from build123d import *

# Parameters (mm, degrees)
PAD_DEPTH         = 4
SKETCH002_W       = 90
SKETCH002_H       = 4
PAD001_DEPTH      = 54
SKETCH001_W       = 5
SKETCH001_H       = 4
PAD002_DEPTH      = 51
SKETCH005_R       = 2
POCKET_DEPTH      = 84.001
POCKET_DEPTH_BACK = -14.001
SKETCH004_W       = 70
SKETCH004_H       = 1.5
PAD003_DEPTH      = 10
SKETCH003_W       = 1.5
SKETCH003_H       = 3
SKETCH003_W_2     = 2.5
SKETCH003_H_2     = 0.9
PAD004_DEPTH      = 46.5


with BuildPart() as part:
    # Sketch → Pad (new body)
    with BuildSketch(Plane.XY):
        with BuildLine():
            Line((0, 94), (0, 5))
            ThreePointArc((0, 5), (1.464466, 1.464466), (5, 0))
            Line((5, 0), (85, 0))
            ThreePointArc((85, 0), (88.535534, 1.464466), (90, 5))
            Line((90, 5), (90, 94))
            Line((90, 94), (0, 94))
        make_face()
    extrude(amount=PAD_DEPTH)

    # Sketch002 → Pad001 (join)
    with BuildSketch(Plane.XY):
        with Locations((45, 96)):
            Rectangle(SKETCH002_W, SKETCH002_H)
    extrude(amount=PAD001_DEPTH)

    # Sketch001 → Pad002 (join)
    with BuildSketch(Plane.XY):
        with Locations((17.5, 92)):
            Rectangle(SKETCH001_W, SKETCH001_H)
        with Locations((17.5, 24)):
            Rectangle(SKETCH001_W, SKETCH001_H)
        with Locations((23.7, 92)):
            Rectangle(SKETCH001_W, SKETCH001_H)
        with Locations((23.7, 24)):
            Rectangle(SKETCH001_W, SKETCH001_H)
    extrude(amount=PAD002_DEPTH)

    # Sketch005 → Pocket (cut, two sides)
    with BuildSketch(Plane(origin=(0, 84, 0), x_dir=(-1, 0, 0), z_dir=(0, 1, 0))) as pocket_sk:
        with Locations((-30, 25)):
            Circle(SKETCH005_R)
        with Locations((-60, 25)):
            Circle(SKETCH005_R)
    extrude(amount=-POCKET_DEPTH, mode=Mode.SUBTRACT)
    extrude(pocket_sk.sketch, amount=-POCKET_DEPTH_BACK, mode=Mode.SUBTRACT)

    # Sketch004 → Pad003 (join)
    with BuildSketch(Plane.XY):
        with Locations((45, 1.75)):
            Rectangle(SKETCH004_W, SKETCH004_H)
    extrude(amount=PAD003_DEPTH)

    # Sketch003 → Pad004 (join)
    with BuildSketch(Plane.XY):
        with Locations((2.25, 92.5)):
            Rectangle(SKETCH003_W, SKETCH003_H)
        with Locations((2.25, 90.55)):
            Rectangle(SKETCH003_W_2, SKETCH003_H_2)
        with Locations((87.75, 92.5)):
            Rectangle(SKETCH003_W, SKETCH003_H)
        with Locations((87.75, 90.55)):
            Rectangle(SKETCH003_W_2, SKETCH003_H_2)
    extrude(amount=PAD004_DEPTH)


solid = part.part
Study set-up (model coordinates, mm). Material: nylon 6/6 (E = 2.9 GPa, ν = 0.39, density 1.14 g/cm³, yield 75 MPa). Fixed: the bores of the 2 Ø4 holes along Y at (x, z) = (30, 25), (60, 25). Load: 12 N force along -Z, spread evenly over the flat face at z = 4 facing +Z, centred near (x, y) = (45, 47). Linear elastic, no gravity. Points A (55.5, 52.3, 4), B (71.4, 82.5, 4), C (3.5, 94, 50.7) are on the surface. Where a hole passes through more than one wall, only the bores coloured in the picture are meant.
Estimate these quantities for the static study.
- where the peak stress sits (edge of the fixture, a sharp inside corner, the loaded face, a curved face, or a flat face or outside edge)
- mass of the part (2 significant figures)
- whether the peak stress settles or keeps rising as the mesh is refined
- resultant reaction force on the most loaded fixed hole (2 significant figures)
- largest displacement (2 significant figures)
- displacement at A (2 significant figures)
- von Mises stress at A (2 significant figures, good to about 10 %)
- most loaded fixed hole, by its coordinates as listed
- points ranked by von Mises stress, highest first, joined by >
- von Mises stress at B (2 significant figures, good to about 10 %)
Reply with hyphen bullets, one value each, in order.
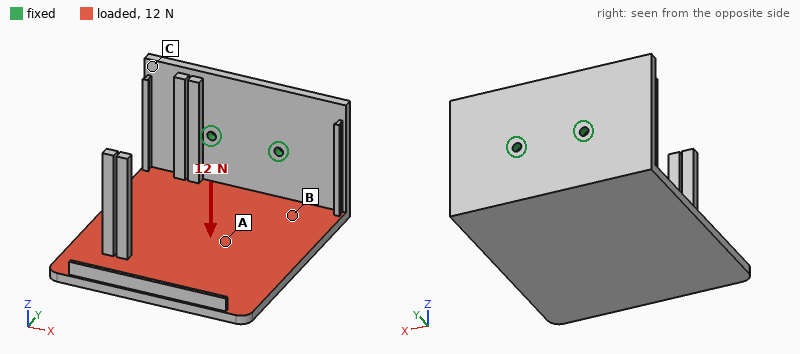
- edge of the fixture
- 66 g
- keeps rising
- 6.8 N
- 1.5 mm
- 0.53 mm
- 0.64 MPa
- (60, 25)
- B > A > C
- 1.4 MPa
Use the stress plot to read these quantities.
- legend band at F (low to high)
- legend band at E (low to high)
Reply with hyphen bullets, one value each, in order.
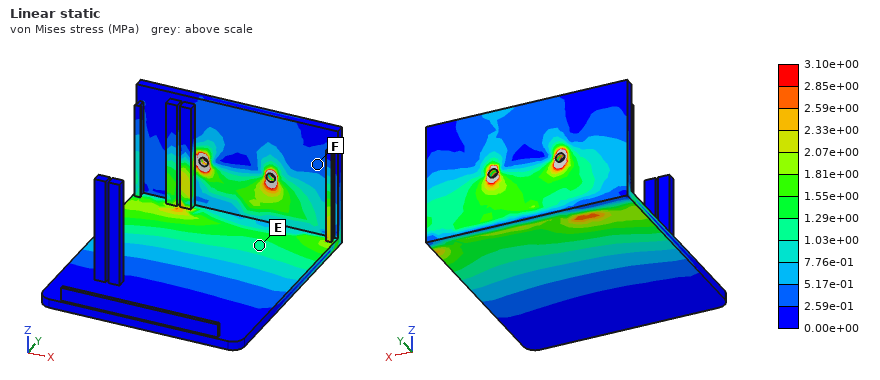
- 2.59e-01 to 5.17e-01 MPa
- 1.03e+00 to 1.29e+00 MPa
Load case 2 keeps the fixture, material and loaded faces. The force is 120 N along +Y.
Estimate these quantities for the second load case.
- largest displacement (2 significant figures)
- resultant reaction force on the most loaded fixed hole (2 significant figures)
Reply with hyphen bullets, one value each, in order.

- 1.4 mm
- 61 N
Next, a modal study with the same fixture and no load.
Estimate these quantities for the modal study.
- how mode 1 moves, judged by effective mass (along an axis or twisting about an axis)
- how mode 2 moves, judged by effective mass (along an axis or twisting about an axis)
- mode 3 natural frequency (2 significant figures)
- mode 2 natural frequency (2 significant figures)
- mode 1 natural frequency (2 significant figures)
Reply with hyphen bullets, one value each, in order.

- along Z
- along X
- 270 Hz
- 180 Hz
- 84 Hz
